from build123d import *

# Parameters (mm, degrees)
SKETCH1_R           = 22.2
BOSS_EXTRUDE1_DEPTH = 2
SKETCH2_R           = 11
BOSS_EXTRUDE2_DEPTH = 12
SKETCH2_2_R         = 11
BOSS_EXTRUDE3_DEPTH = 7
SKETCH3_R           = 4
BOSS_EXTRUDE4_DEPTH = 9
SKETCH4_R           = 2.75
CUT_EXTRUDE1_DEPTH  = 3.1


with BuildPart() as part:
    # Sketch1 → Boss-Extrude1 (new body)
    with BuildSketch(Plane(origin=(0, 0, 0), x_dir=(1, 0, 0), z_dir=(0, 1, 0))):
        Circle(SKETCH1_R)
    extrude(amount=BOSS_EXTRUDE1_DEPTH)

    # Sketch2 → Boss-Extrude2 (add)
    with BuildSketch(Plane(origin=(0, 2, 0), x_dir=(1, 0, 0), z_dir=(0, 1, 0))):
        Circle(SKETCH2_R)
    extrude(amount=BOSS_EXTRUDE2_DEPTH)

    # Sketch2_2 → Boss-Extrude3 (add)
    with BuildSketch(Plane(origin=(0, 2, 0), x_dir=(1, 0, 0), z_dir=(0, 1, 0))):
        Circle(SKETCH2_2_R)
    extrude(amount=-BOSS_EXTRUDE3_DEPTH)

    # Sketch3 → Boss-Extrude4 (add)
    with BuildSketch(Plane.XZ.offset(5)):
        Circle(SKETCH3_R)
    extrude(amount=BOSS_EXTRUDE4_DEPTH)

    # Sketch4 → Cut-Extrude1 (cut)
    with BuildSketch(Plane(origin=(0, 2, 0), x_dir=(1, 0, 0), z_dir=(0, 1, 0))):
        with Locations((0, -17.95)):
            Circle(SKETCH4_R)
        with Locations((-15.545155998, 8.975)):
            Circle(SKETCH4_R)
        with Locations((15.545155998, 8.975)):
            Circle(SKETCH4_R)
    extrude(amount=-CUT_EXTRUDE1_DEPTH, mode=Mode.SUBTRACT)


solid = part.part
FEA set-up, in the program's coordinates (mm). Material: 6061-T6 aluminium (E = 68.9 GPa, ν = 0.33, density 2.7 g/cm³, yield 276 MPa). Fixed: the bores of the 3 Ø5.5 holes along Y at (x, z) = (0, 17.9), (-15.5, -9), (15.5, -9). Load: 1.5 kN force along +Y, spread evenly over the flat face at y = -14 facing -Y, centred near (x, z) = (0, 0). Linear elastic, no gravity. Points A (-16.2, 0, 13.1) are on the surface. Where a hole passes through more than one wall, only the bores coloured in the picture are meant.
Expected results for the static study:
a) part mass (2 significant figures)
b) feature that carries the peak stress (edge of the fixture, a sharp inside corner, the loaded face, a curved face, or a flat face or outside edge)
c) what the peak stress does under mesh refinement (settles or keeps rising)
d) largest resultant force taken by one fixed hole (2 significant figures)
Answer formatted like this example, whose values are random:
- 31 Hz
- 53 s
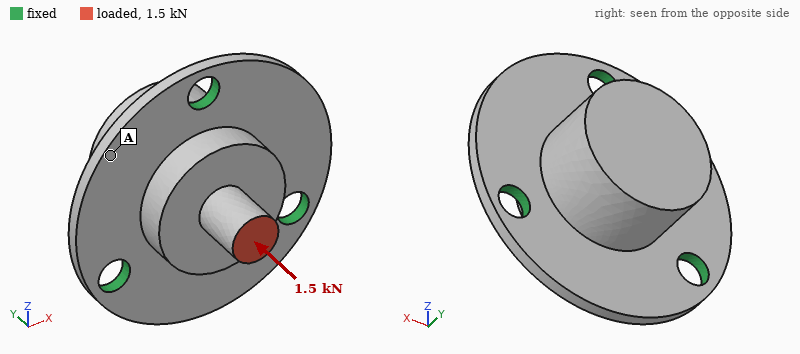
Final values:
- 27 g
- edge of the fixture
- keeps rising
- 500 N
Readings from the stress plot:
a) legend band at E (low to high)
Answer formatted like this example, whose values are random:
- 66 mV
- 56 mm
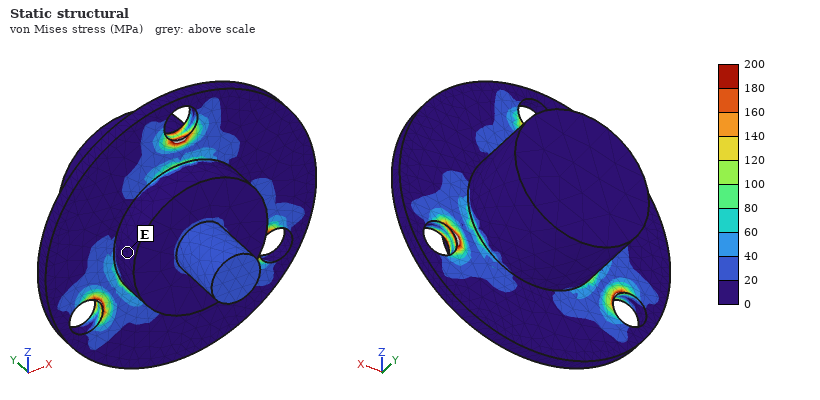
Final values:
- 0 to 20 MPa
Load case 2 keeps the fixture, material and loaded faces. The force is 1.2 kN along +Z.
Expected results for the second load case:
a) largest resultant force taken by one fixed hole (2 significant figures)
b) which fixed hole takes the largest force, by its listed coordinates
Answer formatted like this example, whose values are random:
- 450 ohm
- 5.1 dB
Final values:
- 950 N
- (0, 17.9)
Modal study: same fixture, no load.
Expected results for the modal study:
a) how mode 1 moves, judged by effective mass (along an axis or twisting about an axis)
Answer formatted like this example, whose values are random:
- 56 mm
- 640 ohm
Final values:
- along Y
